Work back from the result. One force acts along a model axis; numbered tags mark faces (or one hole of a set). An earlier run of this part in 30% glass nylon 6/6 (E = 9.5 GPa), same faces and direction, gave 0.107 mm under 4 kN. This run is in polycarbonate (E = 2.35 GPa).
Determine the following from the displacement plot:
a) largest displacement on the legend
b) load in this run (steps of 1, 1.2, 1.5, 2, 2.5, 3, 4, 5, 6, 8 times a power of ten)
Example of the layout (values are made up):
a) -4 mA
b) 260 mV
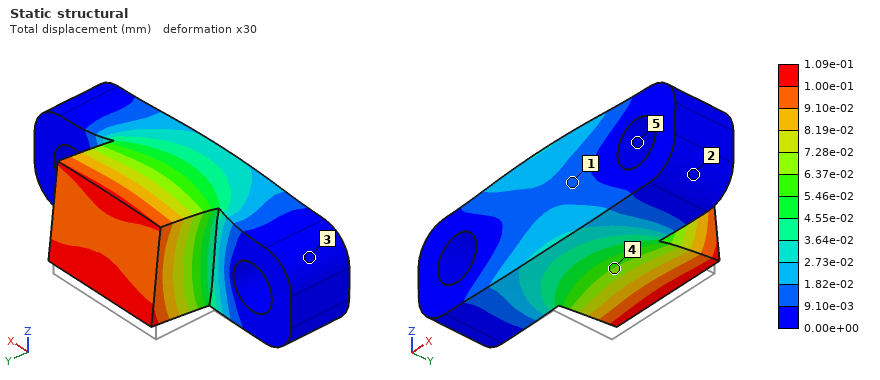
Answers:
a) 1.09e-01 mm
b) 1 kN
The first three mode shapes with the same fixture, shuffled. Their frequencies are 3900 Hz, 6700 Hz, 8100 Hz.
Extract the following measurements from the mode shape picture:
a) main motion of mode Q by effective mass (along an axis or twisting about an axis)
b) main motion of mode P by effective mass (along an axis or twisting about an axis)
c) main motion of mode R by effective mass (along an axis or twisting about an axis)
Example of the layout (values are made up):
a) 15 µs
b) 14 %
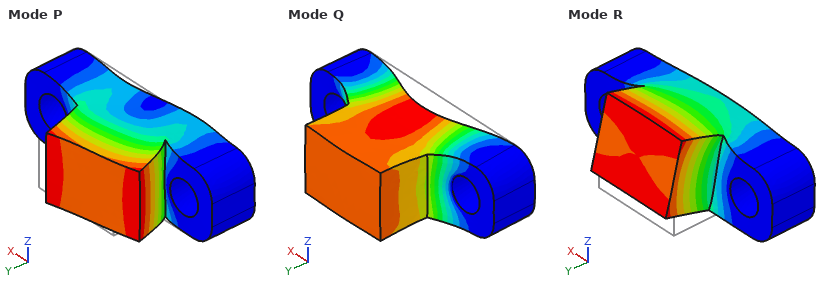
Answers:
a) along Y
b) along X
c) along Z
